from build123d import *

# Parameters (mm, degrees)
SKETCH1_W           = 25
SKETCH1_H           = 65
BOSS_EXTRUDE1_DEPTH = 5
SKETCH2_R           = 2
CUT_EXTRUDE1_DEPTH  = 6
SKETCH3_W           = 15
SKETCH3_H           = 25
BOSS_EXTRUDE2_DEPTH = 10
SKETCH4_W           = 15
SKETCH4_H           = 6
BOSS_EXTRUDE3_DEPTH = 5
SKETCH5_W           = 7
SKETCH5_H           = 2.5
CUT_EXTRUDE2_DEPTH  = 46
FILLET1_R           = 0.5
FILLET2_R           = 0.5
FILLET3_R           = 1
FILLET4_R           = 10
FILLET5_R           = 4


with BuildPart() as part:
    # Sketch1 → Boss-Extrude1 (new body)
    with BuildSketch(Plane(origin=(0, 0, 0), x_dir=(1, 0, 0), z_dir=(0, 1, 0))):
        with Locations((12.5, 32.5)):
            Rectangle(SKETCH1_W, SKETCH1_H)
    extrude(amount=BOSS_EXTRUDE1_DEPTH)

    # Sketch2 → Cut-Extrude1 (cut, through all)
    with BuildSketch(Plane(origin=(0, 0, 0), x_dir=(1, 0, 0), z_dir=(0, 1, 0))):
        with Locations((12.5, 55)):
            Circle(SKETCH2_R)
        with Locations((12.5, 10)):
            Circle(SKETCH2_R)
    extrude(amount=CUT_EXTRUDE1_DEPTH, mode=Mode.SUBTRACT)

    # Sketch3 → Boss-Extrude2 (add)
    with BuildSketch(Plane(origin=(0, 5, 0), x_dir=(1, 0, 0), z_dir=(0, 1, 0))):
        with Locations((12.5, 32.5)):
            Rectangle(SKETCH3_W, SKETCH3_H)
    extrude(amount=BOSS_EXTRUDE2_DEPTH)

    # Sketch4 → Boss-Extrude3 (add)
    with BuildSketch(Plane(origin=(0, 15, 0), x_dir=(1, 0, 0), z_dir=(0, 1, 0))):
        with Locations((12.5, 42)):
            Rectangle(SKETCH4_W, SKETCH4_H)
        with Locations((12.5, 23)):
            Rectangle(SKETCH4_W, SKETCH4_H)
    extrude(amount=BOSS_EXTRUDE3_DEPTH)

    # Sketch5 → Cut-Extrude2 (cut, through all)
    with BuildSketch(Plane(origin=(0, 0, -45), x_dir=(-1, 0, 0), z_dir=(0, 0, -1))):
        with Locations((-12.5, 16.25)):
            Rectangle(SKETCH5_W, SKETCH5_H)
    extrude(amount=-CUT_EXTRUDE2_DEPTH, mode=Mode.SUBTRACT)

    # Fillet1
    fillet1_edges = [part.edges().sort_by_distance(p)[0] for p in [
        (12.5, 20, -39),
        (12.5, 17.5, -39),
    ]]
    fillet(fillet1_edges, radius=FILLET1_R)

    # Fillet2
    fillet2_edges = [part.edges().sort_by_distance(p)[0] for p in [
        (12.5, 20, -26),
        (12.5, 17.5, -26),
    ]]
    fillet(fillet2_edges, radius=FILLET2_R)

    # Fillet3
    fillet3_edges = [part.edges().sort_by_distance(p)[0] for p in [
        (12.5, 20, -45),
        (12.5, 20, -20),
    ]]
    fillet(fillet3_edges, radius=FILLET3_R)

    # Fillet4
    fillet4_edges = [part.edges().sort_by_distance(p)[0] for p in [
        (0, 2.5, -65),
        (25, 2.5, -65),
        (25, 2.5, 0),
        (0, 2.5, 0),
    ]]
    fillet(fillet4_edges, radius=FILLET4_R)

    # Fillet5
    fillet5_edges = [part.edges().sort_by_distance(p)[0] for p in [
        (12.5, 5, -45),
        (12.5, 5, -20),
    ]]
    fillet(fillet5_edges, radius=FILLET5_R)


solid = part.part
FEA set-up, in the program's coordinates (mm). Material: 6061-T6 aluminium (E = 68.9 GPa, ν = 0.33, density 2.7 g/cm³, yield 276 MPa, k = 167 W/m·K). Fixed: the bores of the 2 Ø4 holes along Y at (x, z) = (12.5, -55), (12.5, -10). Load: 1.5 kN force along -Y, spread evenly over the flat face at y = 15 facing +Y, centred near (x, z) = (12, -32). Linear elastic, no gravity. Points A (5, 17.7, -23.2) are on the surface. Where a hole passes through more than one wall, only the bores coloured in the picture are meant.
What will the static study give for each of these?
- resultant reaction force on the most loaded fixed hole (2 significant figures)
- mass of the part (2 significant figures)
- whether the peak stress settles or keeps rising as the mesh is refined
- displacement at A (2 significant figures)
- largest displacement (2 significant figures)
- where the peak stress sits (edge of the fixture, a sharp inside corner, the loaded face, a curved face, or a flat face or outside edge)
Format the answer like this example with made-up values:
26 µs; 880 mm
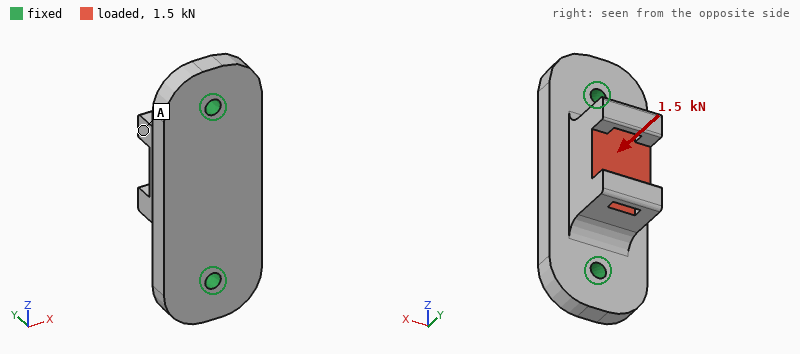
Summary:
860 N; 33 g; keeps rising; 12 µm; 14 µm; edge of the fixture
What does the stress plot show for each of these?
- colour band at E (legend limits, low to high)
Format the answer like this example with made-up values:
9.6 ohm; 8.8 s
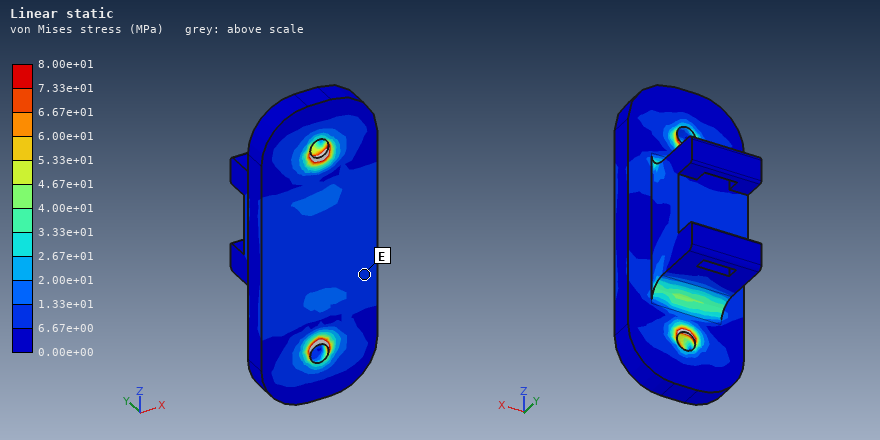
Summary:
6.67e+00 to 1.33e+01 MPa
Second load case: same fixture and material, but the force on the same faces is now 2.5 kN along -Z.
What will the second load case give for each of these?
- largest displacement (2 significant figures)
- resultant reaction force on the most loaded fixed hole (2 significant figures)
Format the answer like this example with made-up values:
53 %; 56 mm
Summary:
17 µm; 1.5 kN
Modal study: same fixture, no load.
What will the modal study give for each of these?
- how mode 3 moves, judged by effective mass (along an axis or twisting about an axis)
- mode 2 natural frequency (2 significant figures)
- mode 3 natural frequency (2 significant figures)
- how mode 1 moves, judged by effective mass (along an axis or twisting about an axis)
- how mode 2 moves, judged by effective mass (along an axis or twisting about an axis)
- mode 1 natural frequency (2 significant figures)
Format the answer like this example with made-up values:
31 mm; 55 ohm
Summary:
along X; 12 kHz; 19 kHz; along X; along Y; 7600 Hz
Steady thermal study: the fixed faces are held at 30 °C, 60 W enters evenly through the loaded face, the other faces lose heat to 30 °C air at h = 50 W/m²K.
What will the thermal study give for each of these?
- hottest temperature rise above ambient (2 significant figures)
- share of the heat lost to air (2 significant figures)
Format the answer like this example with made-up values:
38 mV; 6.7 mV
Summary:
33 K; 6.4 %
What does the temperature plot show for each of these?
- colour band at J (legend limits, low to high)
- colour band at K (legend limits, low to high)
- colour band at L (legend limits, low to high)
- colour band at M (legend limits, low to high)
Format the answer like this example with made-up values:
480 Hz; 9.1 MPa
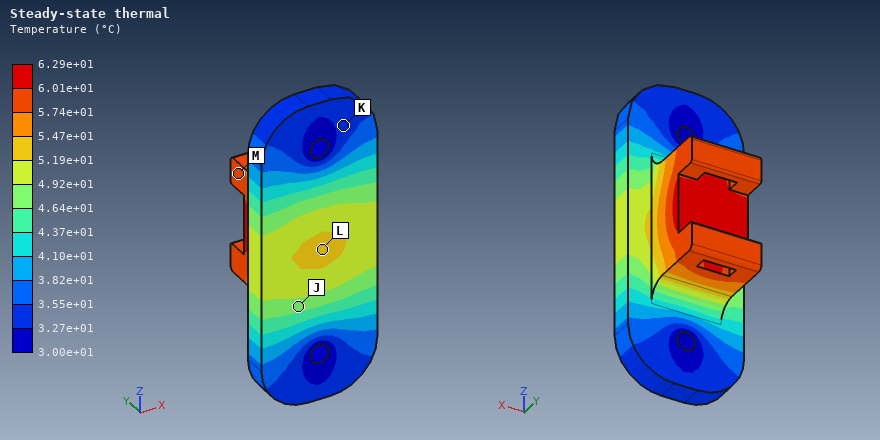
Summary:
4.64e+01 to 4.92e+01 °C; 3.27e+01 to 3.55e+01 °C; 5.19e+01 to 5.47e+01 °C; 5.74e+01 to 6.01e+01 °C
